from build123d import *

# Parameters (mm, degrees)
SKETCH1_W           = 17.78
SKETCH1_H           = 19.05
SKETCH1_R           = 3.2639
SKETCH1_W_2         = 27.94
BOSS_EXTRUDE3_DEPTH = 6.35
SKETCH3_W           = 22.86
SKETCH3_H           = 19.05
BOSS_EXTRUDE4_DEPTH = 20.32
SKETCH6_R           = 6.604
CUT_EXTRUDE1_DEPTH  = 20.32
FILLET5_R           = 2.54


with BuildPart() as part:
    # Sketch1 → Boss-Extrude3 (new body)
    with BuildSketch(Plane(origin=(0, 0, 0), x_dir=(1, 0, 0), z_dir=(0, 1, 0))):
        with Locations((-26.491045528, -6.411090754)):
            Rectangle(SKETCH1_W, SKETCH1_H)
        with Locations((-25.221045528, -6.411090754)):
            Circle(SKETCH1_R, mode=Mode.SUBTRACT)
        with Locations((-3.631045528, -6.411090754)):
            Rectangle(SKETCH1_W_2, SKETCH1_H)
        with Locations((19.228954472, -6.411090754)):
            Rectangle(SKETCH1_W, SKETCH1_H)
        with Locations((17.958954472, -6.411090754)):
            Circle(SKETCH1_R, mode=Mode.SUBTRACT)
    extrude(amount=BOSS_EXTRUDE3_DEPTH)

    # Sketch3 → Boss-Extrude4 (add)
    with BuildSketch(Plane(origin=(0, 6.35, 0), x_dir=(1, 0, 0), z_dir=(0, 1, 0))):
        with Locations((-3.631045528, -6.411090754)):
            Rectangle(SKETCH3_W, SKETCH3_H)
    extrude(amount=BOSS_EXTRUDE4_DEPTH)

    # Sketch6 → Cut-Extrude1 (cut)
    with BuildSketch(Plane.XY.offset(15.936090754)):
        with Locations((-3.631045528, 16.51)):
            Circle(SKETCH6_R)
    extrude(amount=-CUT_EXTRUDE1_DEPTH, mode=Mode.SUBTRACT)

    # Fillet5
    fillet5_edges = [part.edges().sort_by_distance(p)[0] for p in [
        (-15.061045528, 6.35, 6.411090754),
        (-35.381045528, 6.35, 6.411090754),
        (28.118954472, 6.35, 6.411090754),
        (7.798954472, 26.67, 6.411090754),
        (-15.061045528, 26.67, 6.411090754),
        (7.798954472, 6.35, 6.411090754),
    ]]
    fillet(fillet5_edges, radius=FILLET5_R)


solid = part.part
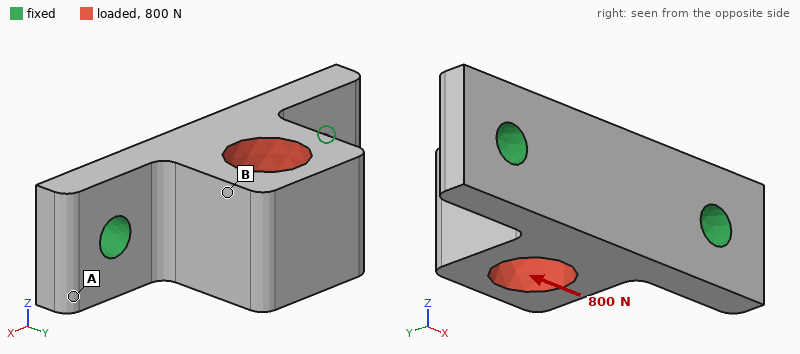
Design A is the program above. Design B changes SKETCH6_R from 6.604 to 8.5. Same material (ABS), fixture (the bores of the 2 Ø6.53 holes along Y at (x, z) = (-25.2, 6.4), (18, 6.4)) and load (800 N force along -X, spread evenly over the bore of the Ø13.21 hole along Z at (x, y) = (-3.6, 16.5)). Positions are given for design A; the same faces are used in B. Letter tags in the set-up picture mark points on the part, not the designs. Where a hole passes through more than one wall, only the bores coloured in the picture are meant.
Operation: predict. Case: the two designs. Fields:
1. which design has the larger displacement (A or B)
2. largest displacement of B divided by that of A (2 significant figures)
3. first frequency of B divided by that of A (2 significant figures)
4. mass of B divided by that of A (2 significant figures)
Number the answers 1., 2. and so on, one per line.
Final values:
1. B
2. 2.2
3. 1.1
4. 0.87
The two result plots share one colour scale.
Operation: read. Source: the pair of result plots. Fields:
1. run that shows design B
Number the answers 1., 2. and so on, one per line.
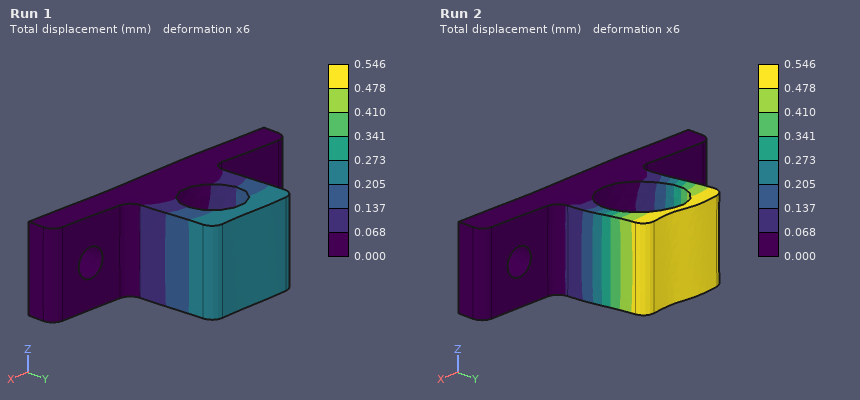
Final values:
1. Run 2
